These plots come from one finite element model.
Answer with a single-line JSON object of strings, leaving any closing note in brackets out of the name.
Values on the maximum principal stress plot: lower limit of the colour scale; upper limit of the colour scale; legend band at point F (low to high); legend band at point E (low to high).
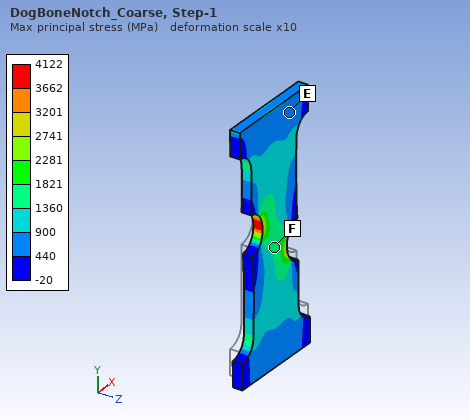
{"lower limit of the colour scale": "-20 MPa", "upper limit of the colour scale": "4122 MPa", "legend band at point F": "1360 to 1821 MPa", "legend band at point E": "440 to 900 MPa"}
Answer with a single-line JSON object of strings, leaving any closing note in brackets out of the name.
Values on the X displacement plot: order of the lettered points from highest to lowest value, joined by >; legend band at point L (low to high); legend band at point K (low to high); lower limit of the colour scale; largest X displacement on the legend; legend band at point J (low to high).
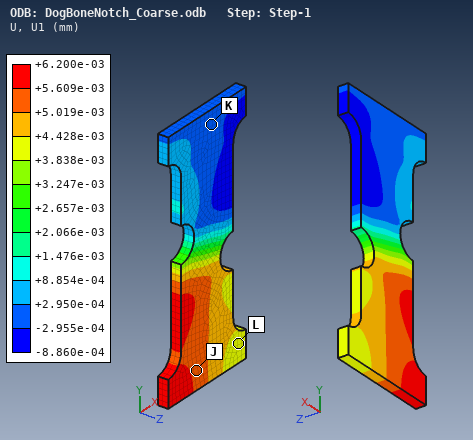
{"order of the lettered points from highest to lowest value, joined by >": "J > L > K", "legend band at point L": "+3.838e-03 to +4.428e-03 mm", "legend band at point K": "-2.955e-04 to +2.950e-04 mm", "lower limit of the colour scale": "-8.860e-04 mm", "largest X displacement on the legend": "+6.200e-03 mm", "legend band at point J": "+5.019e-03 to +5.609e-03 mm"}
